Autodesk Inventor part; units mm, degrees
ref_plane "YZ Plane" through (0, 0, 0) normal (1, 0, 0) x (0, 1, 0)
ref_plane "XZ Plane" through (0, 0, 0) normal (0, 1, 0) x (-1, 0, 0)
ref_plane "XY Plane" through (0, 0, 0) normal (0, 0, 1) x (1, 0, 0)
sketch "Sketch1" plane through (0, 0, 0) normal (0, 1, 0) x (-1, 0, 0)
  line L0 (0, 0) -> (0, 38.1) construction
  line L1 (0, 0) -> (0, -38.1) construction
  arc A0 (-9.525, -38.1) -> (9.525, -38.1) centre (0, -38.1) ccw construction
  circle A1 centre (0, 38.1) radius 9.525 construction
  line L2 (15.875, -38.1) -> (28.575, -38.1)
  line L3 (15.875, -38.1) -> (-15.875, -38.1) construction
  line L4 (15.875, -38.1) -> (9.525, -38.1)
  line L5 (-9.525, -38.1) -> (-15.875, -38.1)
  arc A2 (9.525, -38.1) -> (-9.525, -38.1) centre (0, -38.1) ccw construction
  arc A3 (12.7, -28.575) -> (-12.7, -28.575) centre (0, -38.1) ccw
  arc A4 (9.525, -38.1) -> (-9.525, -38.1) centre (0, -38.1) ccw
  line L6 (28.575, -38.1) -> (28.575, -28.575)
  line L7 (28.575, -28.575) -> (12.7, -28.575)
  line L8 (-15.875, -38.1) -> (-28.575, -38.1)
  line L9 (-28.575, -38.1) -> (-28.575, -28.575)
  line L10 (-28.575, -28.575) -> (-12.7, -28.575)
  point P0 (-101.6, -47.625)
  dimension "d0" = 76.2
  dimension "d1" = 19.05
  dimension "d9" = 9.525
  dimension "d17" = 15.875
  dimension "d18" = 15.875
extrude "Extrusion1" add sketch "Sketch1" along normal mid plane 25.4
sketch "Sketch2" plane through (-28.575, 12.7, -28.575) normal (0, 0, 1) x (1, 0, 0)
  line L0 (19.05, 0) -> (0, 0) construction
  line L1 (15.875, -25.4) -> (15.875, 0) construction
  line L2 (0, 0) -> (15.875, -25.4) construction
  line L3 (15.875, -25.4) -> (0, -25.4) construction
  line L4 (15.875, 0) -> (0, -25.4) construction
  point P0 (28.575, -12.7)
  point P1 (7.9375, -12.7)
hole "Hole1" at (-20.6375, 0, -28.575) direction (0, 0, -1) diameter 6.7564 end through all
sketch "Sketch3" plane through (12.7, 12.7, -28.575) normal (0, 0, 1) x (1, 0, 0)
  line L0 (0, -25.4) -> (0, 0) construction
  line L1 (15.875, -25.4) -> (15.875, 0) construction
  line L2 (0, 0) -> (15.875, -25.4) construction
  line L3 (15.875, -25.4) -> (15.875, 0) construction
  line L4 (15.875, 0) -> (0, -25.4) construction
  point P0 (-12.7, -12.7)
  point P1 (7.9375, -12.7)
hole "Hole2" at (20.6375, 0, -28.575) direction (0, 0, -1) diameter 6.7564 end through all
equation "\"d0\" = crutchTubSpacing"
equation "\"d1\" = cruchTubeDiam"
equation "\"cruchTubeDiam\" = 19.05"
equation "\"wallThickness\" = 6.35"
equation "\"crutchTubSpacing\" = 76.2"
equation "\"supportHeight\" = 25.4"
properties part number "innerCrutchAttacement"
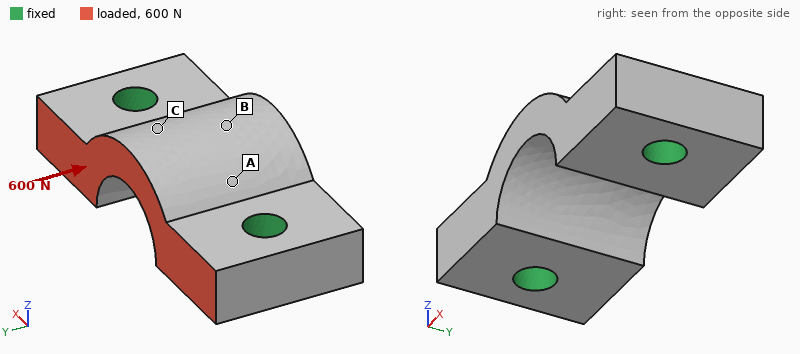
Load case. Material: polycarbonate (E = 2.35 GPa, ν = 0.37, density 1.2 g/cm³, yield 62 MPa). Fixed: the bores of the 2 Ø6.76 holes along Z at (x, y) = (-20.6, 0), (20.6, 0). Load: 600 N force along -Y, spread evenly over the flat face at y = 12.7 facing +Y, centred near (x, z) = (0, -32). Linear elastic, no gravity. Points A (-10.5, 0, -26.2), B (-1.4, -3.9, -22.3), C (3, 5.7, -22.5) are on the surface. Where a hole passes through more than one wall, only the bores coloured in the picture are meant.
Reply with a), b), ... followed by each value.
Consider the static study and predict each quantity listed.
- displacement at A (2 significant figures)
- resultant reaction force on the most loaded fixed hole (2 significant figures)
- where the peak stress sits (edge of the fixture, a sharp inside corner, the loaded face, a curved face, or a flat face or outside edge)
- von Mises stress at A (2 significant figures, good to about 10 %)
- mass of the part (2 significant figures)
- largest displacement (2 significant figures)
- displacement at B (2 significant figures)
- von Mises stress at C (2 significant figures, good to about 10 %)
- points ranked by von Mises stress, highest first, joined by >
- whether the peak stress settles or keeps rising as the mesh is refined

a) 25 µm
b) 300 N
c) edge of the fixture
d) 2.0 MPa
e) 15 g
f) 53 µm
g) 37 µm
h) 1.2 MPa
i) A > C > B
j) keeps rising
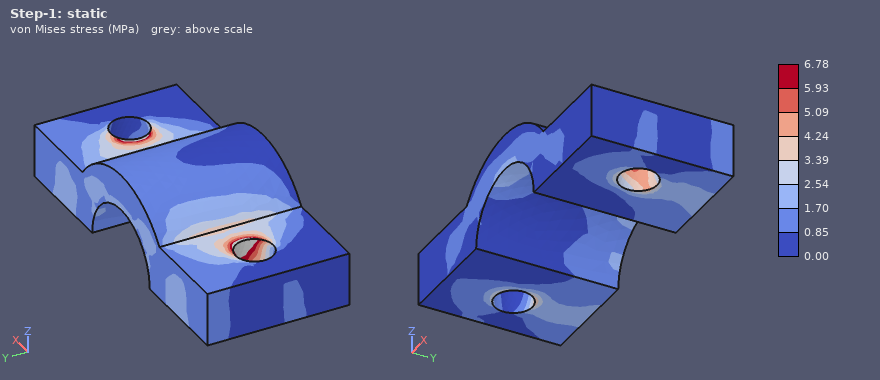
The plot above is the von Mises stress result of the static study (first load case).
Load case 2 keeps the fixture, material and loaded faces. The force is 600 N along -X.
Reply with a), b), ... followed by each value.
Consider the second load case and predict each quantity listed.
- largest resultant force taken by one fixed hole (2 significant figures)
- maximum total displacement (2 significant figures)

a) 320 N
b) 43 µm
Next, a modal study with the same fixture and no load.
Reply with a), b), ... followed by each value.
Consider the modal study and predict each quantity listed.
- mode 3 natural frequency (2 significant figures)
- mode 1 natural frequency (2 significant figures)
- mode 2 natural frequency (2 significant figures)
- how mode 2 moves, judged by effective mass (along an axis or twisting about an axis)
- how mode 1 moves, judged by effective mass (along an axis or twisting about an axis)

a) 9100 Hz
b) 5100 Hz
c) 7400 Hz
d) along Z
e) along Y
